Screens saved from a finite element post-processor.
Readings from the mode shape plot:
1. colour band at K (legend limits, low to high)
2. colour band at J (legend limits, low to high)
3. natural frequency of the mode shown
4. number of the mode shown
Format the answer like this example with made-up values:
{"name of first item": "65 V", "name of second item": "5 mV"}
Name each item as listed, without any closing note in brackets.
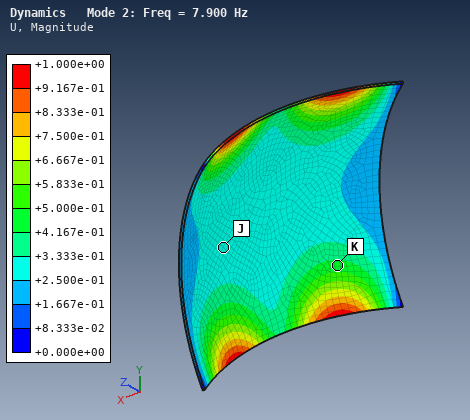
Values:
{"colour band at K": "+4.167e-01 to +5.000e-01", "colour band at J": "+2.500e-01 to +3.333e-01", "natural frequency of the mode shown": "7.900 Hz", "number of the mode shown": "2"}
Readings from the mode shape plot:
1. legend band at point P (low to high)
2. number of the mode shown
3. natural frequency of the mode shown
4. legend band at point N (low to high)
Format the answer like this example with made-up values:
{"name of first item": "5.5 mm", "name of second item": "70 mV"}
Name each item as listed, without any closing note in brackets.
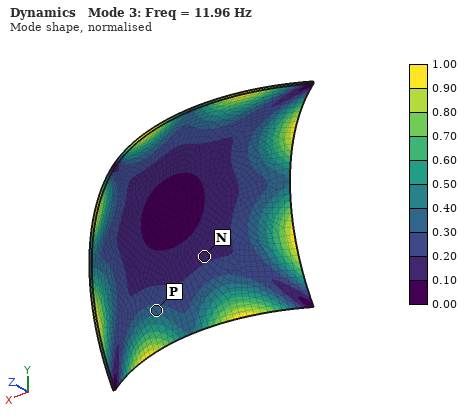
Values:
{"legend band at point P": "0.30 to 0.40", "number of the mode shown": "3", "natural frequency of the mode shown": "11.96 Hz", "legend band at point N": "0.10 to 0.20"}
